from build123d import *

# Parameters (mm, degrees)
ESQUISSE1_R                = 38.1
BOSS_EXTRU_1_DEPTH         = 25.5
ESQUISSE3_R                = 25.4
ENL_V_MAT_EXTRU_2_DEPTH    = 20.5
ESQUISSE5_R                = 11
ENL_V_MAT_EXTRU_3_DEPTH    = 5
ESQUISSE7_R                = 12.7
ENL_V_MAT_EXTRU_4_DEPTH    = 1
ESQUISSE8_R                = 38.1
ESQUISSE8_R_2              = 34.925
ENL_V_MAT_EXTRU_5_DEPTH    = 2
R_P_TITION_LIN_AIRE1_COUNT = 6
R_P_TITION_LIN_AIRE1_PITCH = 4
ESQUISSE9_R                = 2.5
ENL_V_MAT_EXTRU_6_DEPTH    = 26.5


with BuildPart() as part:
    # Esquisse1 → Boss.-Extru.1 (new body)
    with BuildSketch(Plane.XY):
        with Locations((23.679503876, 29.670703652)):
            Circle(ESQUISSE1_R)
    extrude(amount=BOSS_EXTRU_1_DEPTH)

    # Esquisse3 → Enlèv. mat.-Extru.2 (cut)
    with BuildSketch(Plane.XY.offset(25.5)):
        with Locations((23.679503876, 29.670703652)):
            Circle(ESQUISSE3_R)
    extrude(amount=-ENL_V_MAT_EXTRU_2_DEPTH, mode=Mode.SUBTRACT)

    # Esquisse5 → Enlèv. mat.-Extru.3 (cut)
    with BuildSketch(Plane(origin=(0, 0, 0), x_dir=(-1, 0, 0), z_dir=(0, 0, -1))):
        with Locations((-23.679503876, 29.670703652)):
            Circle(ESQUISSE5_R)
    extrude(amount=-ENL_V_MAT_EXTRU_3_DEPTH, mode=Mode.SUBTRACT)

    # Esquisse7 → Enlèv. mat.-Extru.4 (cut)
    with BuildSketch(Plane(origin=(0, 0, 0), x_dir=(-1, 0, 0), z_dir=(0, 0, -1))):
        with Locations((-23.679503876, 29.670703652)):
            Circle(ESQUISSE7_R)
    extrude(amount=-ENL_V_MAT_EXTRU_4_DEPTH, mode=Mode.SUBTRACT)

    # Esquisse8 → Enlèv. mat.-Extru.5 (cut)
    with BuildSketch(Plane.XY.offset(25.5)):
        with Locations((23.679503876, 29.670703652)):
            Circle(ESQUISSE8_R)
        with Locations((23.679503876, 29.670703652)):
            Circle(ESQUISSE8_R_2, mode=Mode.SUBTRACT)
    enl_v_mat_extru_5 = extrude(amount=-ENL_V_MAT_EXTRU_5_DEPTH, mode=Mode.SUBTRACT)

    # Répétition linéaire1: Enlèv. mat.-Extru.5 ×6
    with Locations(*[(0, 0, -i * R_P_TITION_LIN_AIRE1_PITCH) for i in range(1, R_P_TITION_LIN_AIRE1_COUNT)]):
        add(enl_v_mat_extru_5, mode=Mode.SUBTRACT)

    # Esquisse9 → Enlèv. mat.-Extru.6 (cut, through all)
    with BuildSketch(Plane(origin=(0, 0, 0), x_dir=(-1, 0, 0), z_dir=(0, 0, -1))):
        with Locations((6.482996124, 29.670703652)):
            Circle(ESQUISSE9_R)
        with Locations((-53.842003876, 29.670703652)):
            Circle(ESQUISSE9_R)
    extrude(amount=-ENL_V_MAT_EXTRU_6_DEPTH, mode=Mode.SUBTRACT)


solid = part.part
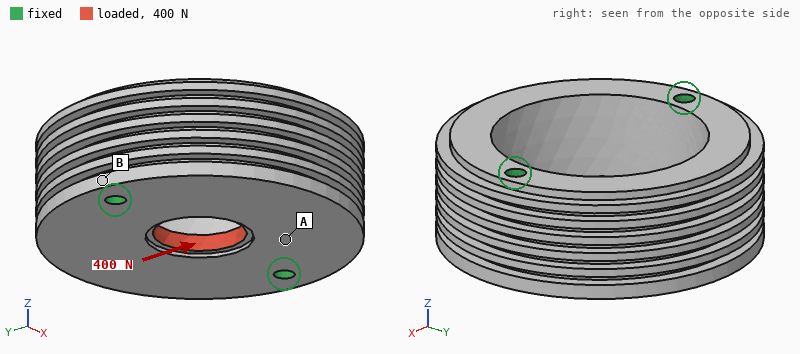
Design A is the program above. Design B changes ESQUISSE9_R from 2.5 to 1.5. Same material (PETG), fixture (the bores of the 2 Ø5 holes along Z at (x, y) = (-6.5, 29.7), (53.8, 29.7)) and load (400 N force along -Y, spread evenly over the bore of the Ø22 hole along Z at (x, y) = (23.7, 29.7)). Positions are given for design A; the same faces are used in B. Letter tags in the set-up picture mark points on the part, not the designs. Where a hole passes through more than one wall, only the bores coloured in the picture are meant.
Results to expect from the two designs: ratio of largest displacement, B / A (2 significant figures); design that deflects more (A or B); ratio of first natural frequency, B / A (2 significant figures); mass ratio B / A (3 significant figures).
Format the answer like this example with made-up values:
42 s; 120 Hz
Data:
1.1; B; 0.92; 1.01
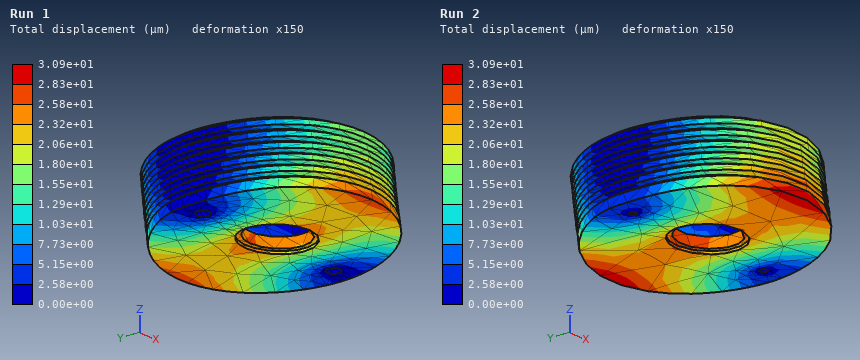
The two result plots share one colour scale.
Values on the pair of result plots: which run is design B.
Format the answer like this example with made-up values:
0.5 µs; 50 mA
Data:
Run 2
